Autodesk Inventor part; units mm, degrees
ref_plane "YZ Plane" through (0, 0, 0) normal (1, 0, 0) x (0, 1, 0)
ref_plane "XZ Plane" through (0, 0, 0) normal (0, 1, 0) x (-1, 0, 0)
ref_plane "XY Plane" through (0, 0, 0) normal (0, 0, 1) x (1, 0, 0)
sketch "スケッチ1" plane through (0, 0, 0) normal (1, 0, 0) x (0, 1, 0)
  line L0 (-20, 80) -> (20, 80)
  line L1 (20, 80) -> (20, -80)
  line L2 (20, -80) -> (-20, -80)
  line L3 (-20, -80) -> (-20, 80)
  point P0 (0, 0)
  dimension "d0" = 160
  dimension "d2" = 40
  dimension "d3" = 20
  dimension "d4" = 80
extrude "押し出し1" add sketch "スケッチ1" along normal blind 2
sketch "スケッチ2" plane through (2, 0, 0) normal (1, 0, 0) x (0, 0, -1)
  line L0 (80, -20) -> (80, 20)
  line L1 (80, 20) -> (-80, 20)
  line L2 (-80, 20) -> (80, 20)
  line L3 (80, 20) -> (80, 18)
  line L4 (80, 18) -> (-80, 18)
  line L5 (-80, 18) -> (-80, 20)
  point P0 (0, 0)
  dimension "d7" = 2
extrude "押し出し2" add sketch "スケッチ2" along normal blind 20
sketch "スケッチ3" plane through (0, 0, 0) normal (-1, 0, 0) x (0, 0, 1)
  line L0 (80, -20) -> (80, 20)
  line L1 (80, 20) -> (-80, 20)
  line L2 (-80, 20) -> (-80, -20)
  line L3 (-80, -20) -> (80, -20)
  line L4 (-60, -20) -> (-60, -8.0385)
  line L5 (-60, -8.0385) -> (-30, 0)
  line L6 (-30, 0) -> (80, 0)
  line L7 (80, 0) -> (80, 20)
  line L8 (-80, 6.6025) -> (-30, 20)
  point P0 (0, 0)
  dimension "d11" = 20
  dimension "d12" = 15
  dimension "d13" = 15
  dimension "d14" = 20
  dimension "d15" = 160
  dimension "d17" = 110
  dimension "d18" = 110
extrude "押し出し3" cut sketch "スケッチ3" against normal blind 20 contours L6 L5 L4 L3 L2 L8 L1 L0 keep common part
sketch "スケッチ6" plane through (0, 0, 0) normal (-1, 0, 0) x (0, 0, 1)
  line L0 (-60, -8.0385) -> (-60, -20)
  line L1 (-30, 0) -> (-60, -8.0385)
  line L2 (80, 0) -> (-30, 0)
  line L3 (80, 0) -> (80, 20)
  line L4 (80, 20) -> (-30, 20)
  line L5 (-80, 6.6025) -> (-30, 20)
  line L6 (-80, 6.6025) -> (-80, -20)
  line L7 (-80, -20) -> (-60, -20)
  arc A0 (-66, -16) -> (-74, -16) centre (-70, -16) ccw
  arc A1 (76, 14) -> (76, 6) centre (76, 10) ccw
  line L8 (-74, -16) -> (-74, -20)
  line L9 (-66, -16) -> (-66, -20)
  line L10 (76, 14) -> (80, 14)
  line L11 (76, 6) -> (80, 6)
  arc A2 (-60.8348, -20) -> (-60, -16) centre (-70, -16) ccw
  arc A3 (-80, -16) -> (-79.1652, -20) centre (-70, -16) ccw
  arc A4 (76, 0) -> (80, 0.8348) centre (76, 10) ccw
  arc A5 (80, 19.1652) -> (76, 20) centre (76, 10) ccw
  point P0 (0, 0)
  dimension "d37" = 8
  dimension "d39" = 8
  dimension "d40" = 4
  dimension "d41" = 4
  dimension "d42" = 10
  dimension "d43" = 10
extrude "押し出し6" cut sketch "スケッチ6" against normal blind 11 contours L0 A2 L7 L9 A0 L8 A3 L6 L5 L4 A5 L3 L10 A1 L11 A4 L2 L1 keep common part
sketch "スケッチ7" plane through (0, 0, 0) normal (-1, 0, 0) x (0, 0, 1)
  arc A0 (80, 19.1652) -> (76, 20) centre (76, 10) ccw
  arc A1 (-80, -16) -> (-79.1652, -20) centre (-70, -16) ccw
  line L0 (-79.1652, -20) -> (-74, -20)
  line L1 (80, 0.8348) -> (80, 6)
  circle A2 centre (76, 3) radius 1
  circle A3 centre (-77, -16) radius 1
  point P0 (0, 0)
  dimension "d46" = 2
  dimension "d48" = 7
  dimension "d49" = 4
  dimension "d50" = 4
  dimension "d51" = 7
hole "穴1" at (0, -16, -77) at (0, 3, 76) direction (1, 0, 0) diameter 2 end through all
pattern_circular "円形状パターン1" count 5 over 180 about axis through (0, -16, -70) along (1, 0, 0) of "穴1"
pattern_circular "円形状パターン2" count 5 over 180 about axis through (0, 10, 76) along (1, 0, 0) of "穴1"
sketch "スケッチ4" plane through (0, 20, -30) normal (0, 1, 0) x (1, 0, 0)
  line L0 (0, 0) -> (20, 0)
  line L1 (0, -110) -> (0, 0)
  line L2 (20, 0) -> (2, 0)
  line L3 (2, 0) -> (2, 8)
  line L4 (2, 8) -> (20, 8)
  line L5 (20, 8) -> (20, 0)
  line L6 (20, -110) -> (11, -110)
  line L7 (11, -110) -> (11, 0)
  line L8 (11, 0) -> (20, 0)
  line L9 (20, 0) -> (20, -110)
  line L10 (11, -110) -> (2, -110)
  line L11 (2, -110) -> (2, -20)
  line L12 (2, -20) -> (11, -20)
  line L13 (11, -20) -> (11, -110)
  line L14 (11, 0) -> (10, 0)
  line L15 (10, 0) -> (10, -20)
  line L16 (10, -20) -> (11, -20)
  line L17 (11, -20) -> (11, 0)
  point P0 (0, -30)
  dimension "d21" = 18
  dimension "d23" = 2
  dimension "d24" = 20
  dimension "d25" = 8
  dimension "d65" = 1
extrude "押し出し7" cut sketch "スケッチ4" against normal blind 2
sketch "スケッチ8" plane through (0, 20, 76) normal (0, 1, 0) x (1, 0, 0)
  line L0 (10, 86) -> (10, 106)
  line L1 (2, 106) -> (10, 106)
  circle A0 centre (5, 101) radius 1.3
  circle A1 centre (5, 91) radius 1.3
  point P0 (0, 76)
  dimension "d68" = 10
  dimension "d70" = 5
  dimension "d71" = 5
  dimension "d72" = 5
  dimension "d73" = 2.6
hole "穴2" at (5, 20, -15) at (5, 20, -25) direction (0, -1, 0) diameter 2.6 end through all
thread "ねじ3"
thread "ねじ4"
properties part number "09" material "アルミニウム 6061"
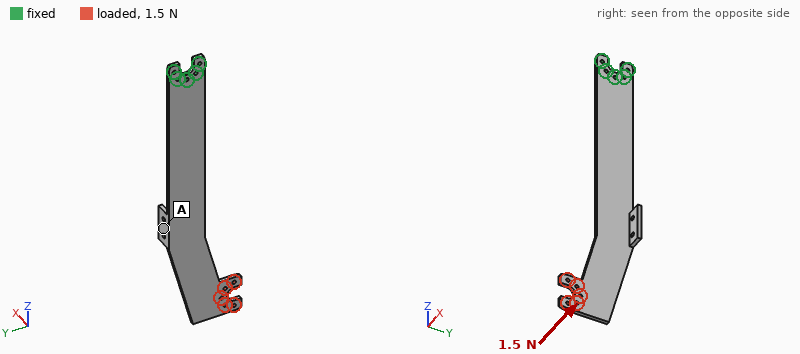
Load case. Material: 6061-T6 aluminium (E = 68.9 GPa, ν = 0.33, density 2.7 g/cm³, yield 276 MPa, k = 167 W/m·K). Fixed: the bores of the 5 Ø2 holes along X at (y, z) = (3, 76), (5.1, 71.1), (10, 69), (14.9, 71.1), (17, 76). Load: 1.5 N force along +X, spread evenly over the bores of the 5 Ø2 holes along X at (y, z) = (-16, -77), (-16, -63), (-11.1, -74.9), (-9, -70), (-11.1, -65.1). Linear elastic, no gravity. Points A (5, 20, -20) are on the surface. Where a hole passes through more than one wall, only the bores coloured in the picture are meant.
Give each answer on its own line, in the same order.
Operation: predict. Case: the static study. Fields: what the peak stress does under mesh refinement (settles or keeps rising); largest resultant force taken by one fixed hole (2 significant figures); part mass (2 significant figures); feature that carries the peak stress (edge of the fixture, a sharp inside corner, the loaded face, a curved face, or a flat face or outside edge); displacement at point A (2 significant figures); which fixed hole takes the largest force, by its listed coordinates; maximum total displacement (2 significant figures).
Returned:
keeps rising
21 N
18 g
edge of the fixture
0.69 mm
(10, 69)
1.7 mm
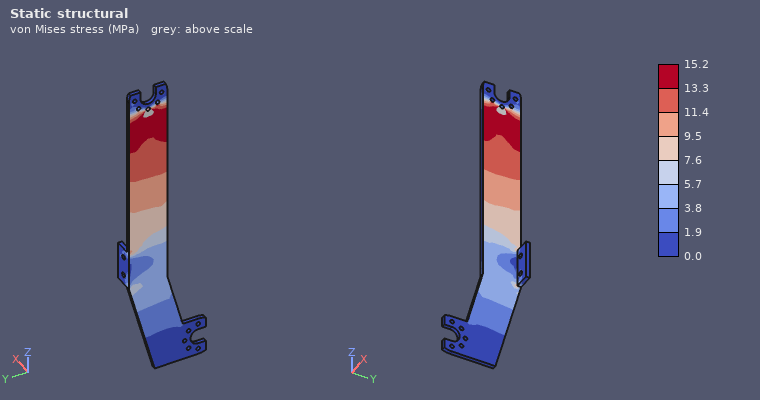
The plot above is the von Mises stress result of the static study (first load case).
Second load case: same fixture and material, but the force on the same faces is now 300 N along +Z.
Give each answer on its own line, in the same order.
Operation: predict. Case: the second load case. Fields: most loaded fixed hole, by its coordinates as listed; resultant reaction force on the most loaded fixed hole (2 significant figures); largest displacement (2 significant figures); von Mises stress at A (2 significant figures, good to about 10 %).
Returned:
(5.1, 71.1)
430 N
0.90 mm
9.5 MPa
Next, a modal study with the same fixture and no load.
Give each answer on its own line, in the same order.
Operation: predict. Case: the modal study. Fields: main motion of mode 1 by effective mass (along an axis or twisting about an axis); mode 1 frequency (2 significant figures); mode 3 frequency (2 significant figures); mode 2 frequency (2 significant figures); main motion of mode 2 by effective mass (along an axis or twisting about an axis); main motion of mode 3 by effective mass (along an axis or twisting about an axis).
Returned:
along X
69 Hz
640 Hz
420 Hz
along X
along Y
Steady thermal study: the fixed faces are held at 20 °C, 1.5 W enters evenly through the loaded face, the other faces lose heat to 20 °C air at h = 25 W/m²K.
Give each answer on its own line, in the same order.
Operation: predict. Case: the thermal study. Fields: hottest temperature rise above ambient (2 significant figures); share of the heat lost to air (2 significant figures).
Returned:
16 K
75 %
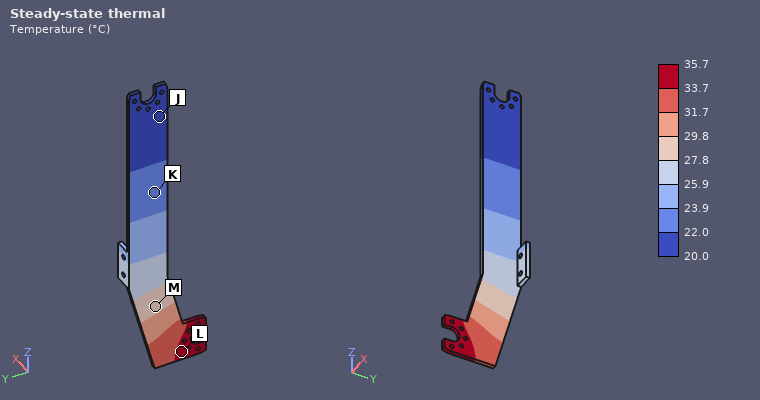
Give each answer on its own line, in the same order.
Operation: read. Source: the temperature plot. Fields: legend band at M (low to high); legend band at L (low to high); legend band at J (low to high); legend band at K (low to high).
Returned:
27.8 to 29.8 °C
33.7 to 35.7 °C
20.0 to 22.0 °C
22.0 to 23.9 °C
